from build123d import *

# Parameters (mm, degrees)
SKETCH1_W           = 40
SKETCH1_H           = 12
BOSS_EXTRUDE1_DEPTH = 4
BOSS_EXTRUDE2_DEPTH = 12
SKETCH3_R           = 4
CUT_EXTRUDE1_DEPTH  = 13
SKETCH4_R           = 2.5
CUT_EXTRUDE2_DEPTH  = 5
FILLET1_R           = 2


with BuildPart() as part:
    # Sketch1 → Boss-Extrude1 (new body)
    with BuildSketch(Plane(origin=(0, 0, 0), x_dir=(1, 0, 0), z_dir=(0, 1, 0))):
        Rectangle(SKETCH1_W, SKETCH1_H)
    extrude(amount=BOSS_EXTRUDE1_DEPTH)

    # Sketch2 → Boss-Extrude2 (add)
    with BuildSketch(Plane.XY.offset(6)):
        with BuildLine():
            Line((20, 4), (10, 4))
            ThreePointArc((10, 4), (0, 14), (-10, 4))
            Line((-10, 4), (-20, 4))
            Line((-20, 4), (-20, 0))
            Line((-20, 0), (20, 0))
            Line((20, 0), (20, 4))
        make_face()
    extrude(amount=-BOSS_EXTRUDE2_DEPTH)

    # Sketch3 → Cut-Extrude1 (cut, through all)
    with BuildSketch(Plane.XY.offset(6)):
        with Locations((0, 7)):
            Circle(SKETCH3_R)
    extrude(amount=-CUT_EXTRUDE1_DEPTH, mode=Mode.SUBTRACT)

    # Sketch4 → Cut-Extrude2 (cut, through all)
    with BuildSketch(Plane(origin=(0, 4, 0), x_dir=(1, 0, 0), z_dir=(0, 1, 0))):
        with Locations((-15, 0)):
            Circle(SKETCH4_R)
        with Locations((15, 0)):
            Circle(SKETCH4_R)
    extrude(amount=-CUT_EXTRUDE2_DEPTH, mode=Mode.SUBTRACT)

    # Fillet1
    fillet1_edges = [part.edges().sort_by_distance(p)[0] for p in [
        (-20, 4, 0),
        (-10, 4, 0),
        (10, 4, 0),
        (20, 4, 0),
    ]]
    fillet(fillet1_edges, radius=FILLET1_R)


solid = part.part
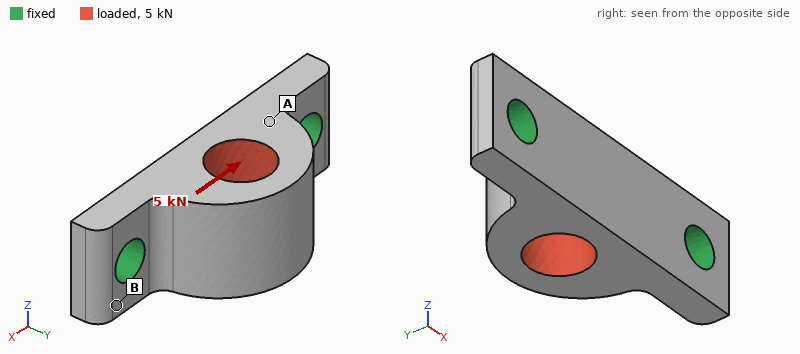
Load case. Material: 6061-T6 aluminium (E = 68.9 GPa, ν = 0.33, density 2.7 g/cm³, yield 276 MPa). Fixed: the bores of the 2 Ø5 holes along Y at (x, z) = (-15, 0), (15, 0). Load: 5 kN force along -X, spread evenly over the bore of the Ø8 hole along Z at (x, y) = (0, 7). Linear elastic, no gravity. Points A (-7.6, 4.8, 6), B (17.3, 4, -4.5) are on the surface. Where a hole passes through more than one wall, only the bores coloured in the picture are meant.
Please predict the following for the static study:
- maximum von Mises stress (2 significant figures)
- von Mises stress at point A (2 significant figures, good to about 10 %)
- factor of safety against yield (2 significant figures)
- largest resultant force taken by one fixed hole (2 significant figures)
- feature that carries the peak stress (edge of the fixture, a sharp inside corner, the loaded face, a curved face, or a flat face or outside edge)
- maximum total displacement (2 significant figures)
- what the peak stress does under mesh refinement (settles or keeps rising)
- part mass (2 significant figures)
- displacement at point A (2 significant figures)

200 MPa
35 MPa
1.4
2.7 kN
a curved face
20 µm
settles
8.2 g
6.8 µm
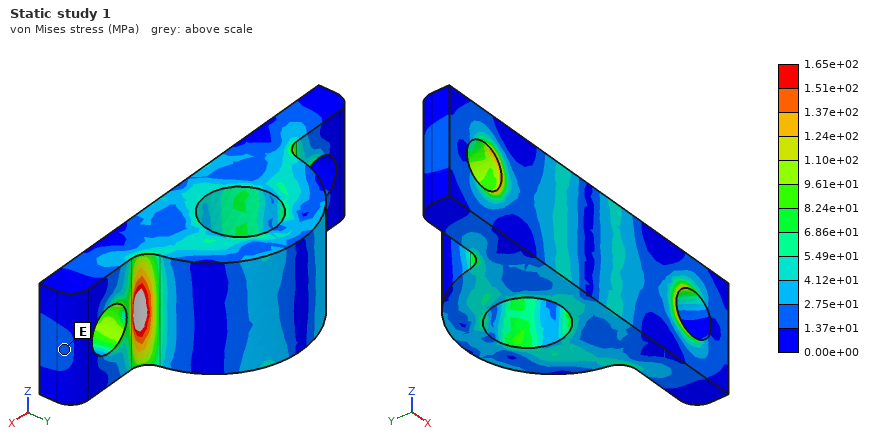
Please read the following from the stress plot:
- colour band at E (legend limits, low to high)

1.37e+01 to 2.75e+01 MPa
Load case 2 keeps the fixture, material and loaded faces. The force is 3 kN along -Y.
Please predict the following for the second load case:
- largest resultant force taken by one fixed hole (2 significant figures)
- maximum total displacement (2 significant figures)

1.6 kN
23 µm
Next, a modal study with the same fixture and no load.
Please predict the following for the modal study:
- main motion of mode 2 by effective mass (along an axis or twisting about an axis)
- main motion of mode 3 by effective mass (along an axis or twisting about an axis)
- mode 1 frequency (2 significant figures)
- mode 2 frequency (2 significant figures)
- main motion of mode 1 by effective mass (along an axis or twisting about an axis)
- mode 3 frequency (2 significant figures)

along Y
along Z
16 kHz
28 kHz
along Z
37 kHz
